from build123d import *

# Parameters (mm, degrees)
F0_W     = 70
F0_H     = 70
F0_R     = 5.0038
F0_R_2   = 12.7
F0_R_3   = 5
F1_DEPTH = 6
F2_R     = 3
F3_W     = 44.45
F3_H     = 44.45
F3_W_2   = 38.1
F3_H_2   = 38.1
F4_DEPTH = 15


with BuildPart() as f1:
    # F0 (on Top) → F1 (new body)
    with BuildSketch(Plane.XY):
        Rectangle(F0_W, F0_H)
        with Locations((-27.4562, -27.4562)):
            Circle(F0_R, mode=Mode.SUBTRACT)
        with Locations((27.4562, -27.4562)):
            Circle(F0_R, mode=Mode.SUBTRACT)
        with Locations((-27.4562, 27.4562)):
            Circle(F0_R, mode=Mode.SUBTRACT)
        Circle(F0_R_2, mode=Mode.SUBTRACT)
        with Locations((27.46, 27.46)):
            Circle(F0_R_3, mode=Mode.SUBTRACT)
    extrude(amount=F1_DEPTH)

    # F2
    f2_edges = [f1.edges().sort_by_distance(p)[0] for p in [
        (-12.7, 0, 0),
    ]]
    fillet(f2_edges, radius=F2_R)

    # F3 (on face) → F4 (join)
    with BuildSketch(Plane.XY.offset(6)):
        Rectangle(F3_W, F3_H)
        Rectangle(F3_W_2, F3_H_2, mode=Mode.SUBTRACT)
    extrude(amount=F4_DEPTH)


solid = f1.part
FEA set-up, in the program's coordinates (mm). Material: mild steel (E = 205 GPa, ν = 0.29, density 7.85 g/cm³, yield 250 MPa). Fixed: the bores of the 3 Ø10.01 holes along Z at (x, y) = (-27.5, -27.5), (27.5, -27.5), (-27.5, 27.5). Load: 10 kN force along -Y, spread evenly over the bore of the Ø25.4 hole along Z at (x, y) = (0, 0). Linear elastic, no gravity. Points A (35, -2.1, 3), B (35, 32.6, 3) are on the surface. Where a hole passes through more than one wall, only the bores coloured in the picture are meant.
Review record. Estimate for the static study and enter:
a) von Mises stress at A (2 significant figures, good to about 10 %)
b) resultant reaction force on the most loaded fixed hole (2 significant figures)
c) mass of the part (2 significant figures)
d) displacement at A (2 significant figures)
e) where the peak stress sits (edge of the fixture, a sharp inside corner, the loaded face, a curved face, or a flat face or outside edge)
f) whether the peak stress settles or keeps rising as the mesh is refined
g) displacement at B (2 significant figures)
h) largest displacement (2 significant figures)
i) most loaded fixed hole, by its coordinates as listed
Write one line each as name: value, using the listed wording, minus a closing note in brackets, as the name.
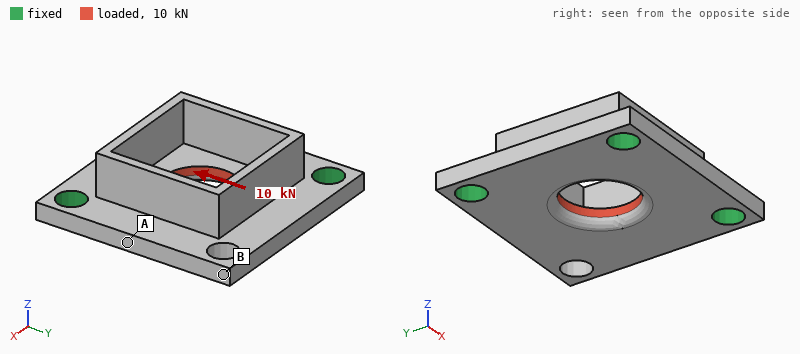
von Mises stress at A: 16 MPa
resultant reaction force on the most loaded fixed hole: 4.5 kN
mass of the part: 250 g
displacement at A: 4.6 µm
where the peak stress sits: edge of the fixture
whether the peak stress settles or keeps rising as the mesh is refined: keeps rising
displacement at B: 11 µm
largest displacement: 11 µm
most loaded fixed hole, by its coordinates as listed: (27.5, -27.5)
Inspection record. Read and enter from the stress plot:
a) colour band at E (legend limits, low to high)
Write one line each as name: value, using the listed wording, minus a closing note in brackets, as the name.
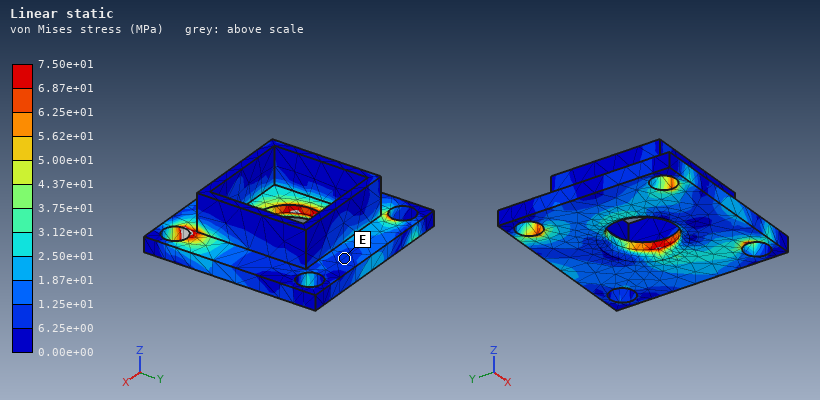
colour band at E: 6.25e+00 to 1.25e+01 MPa
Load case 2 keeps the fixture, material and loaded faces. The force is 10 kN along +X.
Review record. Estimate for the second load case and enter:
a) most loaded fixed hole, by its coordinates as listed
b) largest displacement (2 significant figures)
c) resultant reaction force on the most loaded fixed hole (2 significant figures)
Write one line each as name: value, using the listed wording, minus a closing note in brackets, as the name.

most loaded fixed hole, by its coordinates as listed: (-27.5, 27.5)
largest displacement: 11 µm
resultant reaction force on the most loaded fixed hole: 4.5 kN
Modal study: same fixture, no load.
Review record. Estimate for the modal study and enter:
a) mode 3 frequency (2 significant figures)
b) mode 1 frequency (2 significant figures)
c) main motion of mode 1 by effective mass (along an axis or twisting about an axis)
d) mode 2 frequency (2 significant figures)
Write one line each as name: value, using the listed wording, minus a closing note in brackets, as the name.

mode 3 frequency: 12 kHz
mode 1 frequency: 2900 Hz
main motion of mode 1 by effective mass: along Z
mode 2 frequency: 12 kHz
